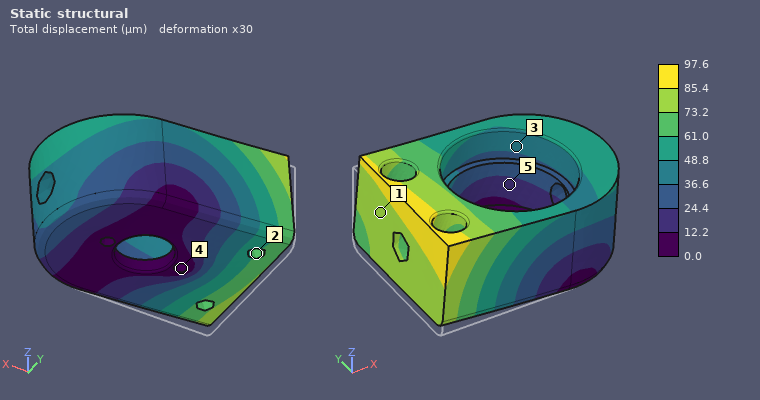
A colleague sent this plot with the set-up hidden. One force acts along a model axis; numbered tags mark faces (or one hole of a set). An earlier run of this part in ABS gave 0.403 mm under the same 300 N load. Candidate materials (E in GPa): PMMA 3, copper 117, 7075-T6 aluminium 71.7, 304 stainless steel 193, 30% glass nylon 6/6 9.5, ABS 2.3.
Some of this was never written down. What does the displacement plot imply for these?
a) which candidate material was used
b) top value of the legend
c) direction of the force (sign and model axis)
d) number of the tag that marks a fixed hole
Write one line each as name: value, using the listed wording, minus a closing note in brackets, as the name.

which candidate material was used: 30% glass nylon 6/6
top value of the legend: 97.6 µm
direction of the force: +Z
number of the tag that marks a fixed hole: 4
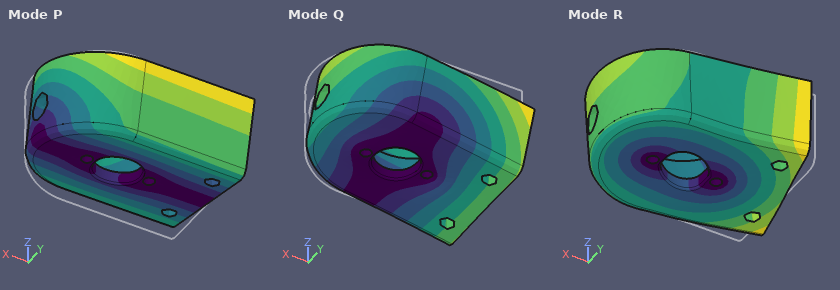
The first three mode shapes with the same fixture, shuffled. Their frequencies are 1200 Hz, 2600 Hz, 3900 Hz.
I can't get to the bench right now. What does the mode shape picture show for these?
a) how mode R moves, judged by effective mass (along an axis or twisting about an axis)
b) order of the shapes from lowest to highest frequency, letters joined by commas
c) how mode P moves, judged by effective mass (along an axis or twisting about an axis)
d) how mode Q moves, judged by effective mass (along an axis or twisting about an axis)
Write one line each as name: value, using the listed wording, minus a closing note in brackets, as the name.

how mode R moves, judged by effective mass: twisting about Z
order of the shapes from lowest to highest frequency, letters joined by commas: P, Q, R
how mode P moves, judged by effective mass: along Y
how mode Q moves, judged by effective mass: along X
